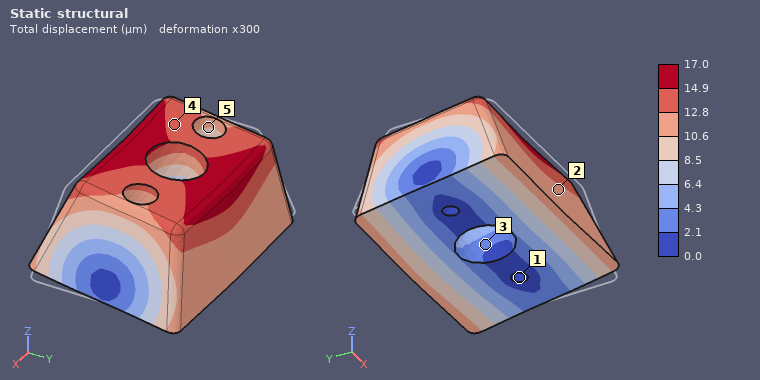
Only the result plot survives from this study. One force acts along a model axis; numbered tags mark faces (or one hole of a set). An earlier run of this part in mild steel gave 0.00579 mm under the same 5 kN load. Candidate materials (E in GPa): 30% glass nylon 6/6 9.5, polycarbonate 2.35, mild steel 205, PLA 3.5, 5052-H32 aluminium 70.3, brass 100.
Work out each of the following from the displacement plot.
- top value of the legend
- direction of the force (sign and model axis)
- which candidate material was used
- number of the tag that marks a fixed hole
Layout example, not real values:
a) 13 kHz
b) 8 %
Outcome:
a) 17.0 µm
b) +Y
c) 5052-H32 aluminium
d) 1
